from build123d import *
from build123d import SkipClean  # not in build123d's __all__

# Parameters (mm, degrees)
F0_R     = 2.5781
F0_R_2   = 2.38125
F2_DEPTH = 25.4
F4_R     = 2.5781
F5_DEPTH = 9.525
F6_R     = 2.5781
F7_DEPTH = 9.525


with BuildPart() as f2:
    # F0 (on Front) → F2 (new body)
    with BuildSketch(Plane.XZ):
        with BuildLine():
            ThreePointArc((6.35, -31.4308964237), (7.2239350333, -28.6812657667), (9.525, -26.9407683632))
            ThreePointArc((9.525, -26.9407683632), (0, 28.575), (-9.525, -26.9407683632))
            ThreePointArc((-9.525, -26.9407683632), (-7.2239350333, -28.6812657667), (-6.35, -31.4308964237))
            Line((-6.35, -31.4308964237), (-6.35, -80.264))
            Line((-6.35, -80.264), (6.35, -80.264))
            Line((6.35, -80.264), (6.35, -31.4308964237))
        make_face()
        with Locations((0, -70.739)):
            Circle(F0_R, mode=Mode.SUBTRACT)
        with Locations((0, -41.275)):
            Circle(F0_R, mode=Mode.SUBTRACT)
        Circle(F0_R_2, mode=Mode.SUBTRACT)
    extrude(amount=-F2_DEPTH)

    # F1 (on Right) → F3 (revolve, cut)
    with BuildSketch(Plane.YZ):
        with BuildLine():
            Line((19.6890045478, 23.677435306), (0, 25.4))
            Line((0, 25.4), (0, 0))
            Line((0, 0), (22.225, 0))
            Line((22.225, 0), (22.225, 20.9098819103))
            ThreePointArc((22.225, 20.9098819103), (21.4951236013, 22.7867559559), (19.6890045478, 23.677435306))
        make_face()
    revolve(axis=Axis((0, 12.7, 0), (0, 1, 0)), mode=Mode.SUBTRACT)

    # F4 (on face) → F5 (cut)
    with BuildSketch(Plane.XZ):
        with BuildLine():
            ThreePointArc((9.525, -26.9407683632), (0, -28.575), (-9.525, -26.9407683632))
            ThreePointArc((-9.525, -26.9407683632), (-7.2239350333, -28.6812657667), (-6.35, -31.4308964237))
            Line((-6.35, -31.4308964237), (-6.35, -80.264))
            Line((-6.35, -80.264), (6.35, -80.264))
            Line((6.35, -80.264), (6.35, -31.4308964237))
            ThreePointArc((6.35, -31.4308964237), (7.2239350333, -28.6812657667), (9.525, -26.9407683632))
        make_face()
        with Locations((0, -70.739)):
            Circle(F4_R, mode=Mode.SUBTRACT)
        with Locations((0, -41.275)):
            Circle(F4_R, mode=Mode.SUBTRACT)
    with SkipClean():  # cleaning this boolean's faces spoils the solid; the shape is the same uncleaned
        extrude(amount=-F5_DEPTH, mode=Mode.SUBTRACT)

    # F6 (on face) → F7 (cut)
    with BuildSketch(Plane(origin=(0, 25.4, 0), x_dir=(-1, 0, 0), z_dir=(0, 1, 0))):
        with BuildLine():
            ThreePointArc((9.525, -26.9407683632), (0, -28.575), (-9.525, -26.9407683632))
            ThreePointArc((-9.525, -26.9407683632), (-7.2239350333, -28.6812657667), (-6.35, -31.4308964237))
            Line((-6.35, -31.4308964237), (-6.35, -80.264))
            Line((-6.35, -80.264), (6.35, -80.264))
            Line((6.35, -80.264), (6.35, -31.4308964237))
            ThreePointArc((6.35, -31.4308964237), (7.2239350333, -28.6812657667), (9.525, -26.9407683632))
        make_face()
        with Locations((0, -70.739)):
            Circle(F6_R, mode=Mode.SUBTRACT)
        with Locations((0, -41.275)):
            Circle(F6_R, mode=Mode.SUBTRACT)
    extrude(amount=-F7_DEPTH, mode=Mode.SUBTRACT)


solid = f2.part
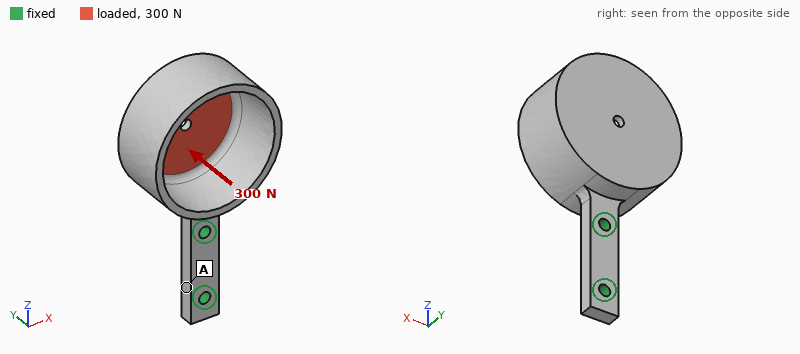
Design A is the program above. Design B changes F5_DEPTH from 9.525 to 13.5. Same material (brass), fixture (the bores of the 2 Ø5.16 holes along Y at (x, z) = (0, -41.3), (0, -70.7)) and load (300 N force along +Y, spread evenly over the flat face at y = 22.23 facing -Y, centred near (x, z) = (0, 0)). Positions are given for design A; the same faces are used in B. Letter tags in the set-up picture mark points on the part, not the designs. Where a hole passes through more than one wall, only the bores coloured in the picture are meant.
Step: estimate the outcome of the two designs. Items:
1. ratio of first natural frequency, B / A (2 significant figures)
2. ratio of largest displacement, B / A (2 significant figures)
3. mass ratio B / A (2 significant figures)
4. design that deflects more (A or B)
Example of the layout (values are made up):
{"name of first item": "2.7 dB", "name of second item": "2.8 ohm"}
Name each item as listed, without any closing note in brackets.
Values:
{"ratio of first natural frequency, B / A": "0.27", "ratio of largest displacement, B / A": "14", "mass ratio B / A": "0.91", "design that deflects more": "B"}
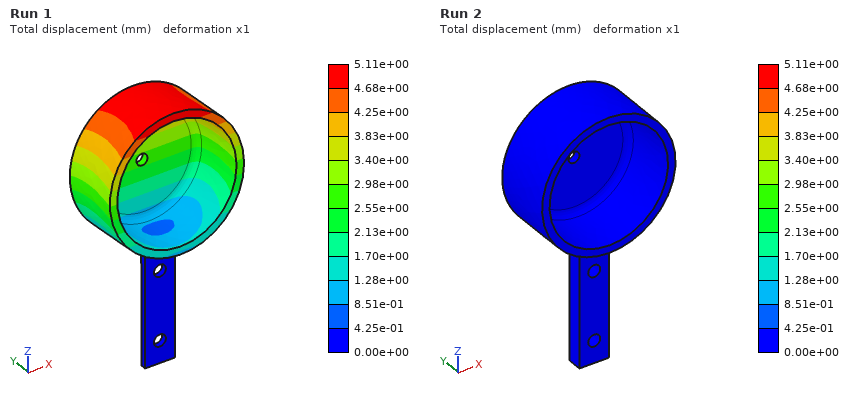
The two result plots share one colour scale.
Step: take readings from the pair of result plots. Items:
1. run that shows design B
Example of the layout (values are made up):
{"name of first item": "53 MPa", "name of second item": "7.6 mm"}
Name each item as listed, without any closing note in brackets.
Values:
{"run that shows design B": "Run 1"}
